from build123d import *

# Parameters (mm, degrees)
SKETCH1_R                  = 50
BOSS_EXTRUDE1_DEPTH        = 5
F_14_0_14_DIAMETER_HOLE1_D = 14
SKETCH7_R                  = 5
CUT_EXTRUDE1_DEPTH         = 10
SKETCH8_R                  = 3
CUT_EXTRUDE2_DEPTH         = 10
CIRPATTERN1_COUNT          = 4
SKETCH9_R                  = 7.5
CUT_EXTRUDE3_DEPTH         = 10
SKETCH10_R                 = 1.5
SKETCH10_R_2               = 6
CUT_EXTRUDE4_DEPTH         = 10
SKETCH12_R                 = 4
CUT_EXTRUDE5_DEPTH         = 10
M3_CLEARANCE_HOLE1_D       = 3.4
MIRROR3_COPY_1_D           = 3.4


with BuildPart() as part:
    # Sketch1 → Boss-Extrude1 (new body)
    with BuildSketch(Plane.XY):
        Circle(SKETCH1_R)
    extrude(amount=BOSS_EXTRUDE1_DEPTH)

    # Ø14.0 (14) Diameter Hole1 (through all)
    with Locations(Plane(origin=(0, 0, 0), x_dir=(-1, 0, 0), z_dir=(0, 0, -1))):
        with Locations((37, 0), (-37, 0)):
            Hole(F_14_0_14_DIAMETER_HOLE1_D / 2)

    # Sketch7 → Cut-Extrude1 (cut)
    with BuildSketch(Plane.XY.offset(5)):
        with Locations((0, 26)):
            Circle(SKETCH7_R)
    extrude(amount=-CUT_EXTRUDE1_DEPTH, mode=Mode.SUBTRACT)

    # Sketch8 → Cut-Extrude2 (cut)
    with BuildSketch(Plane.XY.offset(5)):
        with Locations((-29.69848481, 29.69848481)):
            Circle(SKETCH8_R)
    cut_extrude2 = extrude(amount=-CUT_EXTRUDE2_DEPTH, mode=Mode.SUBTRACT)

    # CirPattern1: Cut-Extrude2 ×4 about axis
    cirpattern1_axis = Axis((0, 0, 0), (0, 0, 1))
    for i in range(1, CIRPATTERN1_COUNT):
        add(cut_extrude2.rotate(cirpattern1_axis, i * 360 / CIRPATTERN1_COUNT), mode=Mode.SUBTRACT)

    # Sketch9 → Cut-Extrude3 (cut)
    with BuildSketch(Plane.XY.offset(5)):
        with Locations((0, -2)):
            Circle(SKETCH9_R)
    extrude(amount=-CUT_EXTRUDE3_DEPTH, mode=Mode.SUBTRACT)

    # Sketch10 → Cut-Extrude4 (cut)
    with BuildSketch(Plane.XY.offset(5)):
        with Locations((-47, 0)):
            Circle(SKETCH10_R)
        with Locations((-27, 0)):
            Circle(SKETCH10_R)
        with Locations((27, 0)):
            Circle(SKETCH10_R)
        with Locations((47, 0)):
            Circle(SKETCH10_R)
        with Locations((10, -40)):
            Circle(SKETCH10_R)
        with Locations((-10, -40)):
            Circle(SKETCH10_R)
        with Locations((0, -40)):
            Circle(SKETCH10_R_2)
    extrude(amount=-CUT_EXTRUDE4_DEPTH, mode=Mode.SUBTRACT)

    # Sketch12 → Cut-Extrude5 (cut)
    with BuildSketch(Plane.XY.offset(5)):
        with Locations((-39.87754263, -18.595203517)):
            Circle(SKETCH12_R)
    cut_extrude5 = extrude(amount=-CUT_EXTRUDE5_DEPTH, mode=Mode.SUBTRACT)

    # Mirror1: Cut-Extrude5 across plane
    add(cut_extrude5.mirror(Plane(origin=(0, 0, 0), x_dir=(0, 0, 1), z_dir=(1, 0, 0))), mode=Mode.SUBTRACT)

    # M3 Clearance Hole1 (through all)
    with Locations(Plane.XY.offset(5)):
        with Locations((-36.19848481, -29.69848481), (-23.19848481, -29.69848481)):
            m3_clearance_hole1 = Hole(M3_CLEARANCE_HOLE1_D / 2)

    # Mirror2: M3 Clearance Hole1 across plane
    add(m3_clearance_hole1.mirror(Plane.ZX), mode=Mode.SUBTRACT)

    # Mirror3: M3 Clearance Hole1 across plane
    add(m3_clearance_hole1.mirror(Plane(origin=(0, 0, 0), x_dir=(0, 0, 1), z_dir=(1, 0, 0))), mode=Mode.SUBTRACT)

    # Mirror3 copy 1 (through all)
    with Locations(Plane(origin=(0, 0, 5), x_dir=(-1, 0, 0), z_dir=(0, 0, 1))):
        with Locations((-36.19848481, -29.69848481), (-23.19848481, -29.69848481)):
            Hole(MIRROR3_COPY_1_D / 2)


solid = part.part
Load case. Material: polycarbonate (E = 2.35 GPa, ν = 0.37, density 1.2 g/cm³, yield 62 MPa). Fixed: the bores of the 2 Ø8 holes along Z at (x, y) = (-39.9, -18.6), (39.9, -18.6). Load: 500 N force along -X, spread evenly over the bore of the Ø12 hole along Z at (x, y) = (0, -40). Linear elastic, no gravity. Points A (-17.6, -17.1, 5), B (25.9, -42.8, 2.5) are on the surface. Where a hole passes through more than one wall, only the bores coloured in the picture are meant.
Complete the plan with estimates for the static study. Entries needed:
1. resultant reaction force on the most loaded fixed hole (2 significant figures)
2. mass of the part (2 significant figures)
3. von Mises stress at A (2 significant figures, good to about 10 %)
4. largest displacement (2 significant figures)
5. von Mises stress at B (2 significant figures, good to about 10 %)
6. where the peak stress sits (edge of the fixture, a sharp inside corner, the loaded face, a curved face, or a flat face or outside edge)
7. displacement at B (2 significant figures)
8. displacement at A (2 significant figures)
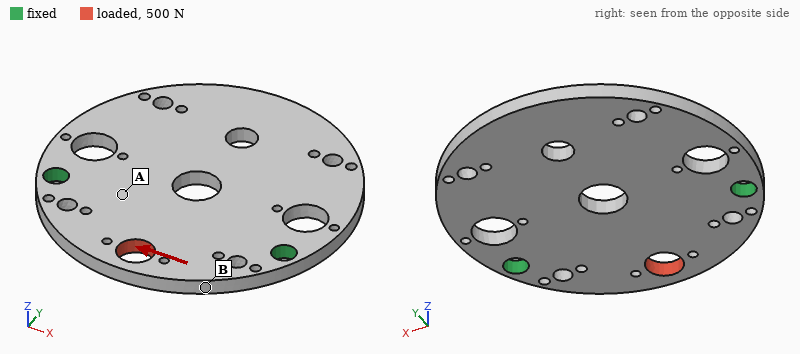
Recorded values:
280 N
41 g
1.2 MPa
88 µm
2.9 MPa
a curved face
54 µm
17 µm
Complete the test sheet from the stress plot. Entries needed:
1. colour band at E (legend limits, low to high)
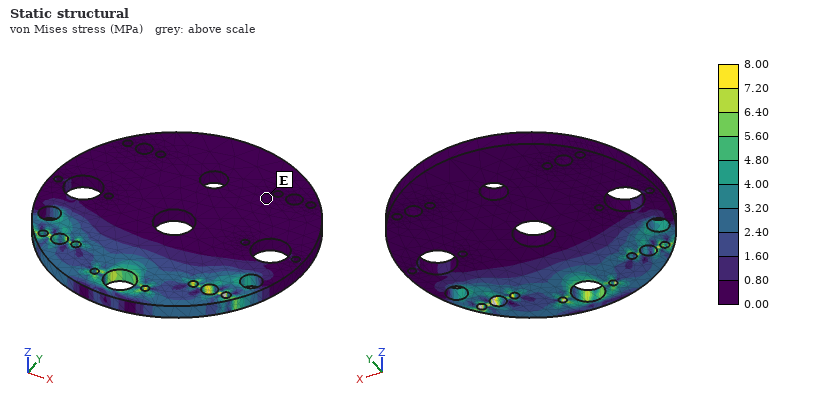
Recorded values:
0.00 to 0.80 MPa
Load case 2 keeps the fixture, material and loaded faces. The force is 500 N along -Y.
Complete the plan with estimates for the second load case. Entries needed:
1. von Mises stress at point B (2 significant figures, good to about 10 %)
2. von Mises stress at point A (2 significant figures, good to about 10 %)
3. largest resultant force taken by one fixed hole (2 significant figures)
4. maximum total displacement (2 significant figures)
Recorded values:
1.4 MPa
1.6 MPa
260 N
0.11 mm
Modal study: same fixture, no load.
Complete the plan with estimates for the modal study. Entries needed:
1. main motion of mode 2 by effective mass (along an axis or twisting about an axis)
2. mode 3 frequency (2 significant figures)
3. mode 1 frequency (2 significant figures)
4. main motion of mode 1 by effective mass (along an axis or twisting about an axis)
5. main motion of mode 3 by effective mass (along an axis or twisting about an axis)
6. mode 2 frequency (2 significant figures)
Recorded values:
twisting about Y
840 Hz
230 Hz
along Z
along Z
660 Hz
